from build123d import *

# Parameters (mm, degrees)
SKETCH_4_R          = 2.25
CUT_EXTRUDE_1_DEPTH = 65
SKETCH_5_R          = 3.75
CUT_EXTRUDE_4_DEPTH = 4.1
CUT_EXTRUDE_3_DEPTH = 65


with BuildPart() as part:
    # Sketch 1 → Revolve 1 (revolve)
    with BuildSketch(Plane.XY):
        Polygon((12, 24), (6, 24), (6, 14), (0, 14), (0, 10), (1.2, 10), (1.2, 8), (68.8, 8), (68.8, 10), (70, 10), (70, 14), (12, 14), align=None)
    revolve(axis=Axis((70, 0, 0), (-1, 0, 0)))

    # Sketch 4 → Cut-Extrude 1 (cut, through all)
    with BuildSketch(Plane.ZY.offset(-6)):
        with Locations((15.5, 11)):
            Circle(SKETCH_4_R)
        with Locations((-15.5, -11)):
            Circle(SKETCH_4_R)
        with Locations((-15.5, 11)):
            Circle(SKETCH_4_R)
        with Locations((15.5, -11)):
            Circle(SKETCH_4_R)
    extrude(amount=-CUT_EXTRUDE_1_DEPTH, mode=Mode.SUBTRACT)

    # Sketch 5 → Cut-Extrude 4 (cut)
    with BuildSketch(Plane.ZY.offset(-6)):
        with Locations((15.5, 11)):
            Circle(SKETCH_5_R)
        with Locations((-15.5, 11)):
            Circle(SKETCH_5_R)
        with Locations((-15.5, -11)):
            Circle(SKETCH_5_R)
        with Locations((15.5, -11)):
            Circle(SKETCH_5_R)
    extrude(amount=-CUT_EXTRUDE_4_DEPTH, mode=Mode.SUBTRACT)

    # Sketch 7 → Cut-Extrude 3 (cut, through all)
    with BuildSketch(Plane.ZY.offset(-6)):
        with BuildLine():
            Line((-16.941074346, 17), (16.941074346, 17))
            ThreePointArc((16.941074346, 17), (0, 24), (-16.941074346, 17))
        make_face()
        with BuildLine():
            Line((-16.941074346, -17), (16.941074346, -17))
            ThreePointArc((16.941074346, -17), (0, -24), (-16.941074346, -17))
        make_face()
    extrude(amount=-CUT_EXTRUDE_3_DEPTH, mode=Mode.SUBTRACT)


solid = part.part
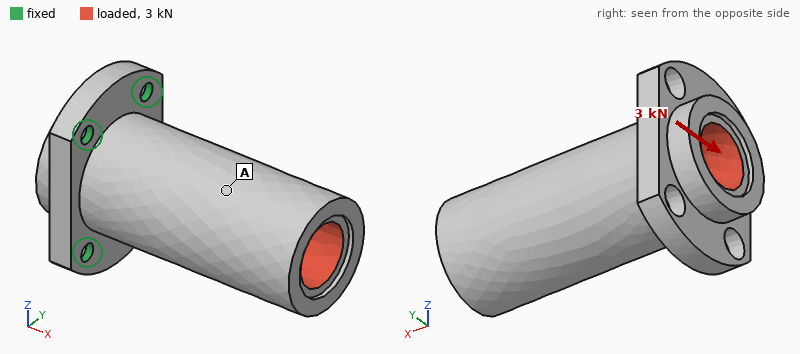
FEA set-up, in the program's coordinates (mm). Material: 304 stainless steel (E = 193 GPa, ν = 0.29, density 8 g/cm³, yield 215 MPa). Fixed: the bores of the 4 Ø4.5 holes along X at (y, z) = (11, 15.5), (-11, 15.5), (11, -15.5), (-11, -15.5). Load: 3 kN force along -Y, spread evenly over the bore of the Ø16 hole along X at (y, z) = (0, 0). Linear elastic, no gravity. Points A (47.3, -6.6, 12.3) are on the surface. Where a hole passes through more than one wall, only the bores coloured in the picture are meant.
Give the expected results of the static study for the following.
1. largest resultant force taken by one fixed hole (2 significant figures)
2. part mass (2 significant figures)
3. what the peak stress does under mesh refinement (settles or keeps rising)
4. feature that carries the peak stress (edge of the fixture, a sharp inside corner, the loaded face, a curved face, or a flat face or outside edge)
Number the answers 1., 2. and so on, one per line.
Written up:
1. 1.8 kN
2. 260 g
3. keeps rising
4. edge of the fixture
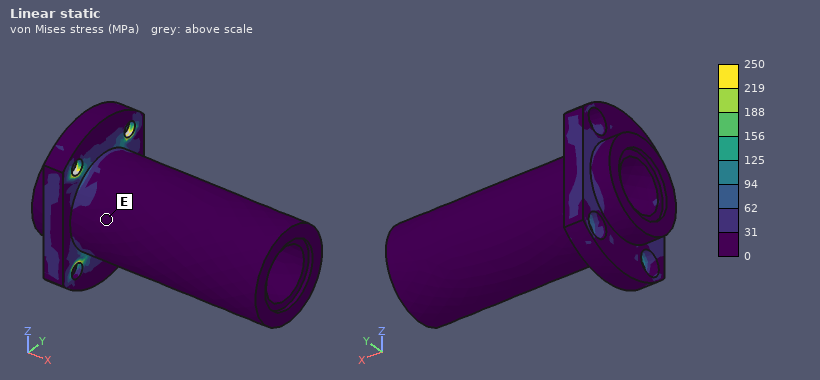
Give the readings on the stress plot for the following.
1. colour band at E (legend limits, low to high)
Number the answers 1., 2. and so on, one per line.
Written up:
1. 0 to 31 MPa
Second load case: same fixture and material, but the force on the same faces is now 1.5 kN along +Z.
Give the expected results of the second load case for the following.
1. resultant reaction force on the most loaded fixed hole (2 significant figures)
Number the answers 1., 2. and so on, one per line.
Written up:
1. 730 N
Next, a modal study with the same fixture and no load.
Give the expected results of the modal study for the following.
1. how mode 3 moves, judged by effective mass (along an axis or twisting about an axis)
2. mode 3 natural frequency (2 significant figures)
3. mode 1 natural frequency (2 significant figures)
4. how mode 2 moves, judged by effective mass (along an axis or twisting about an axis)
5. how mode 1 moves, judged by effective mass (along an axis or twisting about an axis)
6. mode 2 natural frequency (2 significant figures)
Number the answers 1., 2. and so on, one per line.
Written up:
1. along X
2. 10 kHz
3. 2900 Hz
4. along Z
5. along Y
6. 3600 Hz
